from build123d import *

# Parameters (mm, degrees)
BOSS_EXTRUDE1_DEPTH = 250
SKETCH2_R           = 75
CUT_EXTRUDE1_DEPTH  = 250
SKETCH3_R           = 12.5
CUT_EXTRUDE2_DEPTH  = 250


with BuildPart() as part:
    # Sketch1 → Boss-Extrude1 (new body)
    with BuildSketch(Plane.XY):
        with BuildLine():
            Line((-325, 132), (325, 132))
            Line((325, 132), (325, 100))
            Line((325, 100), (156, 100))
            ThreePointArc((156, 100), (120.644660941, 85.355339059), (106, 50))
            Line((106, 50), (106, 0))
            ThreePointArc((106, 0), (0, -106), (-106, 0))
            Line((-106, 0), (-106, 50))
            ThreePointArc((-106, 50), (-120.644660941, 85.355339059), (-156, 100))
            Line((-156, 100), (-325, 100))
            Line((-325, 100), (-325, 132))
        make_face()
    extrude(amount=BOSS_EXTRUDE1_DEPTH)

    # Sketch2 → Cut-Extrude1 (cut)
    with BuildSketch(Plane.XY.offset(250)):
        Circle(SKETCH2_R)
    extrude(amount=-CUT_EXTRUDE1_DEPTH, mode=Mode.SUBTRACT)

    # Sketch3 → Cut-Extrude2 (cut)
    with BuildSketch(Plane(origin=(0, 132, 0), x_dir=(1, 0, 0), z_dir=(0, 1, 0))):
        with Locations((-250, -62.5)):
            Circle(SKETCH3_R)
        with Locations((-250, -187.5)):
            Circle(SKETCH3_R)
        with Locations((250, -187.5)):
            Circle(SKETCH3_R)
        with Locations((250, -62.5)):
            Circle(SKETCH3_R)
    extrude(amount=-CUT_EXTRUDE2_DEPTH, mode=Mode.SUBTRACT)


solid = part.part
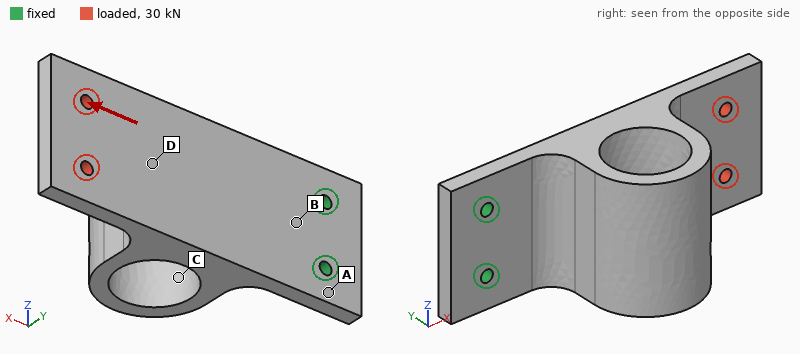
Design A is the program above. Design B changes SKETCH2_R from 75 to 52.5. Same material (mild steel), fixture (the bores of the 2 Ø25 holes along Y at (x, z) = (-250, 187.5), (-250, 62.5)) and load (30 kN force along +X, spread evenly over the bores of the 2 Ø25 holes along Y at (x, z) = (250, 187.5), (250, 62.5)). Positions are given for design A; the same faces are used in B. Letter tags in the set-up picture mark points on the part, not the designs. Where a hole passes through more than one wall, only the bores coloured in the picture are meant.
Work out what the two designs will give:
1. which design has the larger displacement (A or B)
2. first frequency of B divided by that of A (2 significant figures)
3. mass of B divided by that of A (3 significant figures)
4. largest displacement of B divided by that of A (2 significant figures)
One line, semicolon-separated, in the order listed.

A; 0.93; 1.21; 0.88
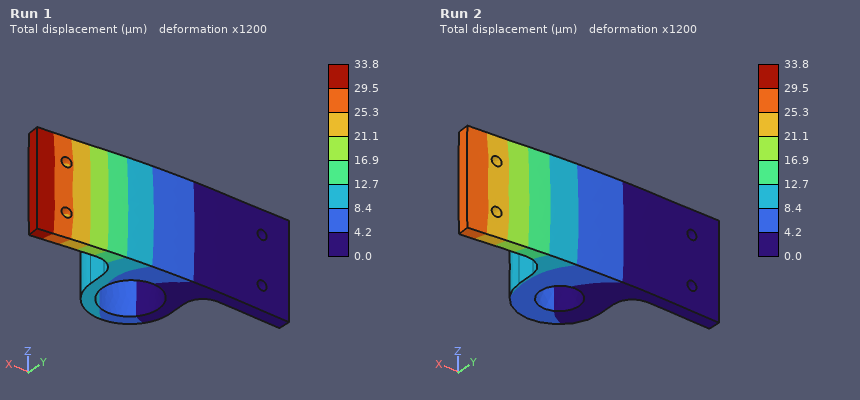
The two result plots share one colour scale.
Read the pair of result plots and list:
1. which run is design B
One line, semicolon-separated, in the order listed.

Run 2
